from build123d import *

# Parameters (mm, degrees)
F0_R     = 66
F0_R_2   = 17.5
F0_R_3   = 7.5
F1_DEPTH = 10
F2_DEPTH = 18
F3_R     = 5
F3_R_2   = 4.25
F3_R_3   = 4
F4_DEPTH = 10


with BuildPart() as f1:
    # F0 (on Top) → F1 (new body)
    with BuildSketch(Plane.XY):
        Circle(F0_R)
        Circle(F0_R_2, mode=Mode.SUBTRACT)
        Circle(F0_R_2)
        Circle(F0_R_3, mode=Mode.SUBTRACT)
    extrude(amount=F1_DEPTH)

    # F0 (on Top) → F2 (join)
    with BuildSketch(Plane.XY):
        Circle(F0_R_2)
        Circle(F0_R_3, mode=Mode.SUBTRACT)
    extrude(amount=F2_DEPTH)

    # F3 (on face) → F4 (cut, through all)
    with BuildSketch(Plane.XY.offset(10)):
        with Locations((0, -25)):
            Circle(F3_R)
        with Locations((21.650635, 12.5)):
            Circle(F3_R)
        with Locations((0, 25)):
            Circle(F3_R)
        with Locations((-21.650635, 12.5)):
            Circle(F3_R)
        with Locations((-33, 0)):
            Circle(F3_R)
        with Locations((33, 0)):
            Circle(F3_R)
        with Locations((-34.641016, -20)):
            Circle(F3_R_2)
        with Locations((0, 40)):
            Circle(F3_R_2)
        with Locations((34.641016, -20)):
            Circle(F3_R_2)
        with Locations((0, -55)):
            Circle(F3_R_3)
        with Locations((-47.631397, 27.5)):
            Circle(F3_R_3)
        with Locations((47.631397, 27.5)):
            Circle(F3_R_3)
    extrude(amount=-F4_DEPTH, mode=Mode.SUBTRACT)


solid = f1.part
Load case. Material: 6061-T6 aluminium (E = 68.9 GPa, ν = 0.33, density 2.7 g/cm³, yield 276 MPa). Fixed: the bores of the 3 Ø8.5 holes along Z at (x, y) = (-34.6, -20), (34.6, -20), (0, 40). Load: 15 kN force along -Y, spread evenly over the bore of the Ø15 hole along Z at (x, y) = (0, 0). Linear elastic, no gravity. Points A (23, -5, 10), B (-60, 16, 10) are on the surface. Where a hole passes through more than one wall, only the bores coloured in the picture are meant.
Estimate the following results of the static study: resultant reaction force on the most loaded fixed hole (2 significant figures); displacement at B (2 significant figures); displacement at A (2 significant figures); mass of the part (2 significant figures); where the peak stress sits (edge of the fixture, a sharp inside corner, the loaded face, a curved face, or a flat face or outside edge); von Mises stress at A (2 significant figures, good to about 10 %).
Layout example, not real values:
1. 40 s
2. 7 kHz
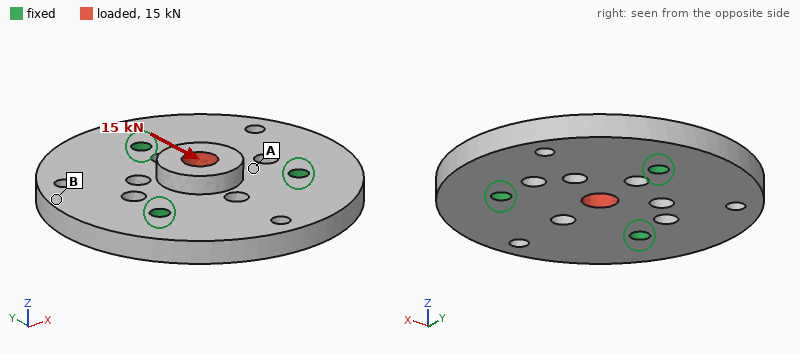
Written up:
1. 5.1 kN
2. 4.1 µm
3. 7.1 µm
4. 360 g
5. a curved face
6. 21 MPa
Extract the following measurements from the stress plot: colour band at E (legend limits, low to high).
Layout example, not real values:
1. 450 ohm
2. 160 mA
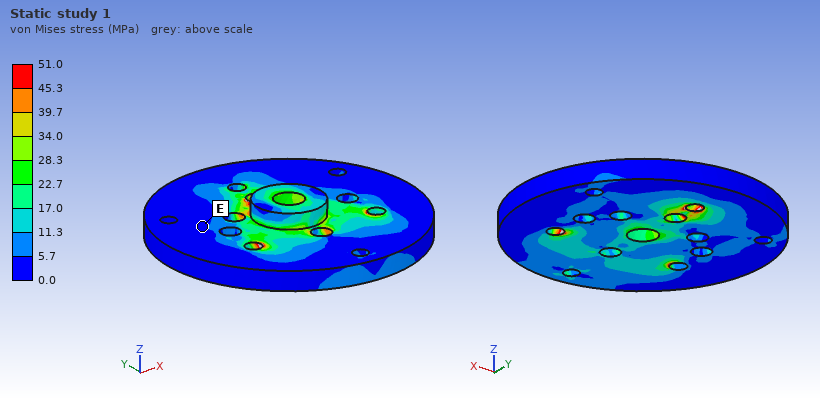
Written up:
1. 0.0 to 5.7 MPa
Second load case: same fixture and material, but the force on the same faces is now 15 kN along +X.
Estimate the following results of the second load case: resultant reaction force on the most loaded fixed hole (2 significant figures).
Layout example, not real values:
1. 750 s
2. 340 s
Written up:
1. 5.6 kN
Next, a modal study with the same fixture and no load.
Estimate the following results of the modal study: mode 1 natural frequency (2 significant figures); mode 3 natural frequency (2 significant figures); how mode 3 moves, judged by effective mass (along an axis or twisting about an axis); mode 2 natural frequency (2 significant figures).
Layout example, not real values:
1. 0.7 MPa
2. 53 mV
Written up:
1. 3900 Hz
2. 4600 Hz
3. along Z
4. 4000 Hz
